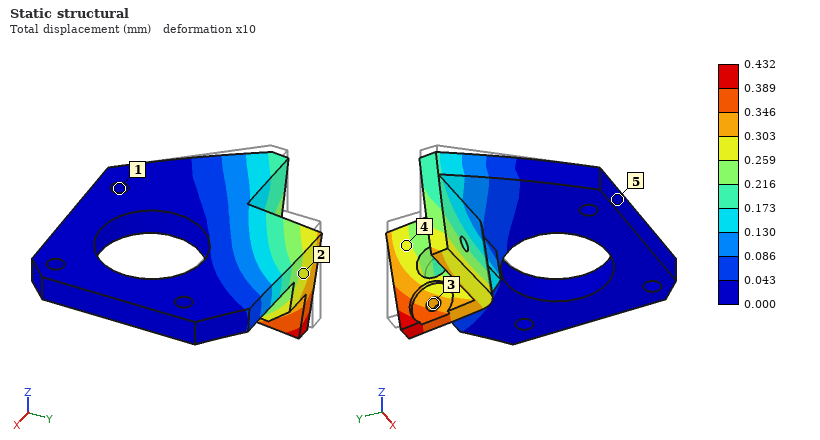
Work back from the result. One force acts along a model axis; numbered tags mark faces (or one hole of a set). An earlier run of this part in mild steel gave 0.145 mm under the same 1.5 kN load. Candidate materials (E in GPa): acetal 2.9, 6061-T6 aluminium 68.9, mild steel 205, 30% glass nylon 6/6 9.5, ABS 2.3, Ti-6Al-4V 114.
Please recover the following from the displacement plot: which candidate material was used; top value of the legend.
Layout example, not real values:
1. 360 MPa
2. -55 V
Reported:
1. 6061-T6 aluminium
2. 0.432 mm
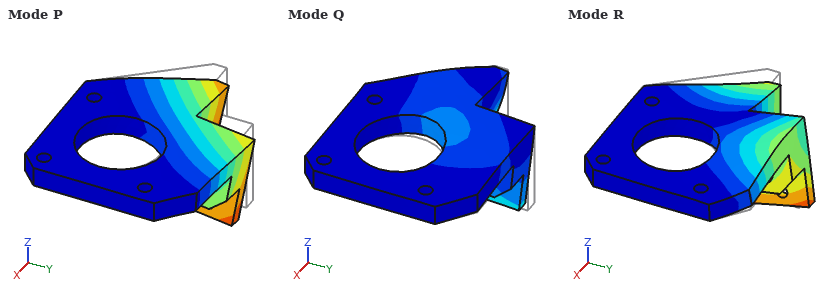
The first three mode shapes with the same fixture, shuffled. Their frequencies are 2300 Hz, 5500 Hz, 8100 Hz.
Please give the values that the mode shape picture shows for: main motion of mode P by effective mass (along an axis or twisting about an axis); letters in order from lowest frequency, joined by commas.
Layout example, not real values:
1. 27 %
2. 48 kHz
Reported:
1. along Z
2. P, R, Q
